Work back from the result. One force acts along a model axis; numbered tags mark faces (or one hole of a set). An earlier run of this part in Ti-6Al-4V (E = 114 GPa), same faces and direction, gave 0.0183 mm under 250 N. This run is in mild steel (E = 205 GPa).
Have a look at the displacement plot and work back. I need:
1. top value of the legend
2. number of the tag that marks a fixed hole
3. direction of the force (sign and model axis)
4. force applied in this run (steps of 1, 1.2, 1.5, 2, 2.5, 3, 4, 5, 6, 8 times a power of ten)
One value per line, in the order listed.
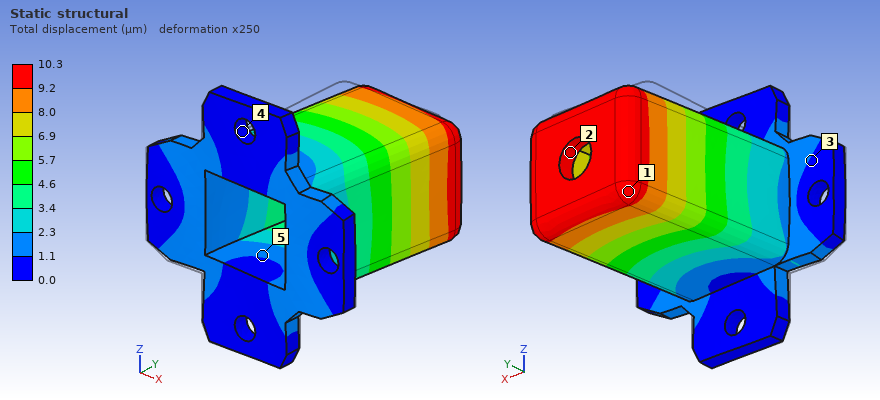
10.3 µm
4
+X
250 N
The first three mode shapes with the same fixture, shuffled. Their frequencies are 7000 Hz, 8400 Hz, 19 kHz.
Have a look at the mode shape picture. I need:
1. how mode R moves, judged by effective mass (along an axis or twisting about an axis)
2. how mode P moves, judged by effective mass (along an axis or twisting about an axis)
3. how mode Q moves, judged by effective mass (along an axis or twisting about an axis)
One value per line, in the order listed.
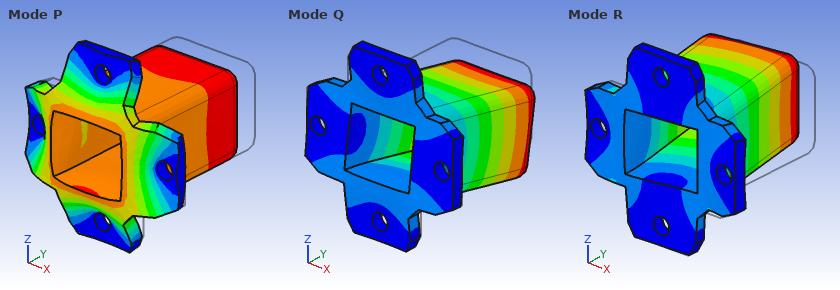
along X
along Y
along Z
